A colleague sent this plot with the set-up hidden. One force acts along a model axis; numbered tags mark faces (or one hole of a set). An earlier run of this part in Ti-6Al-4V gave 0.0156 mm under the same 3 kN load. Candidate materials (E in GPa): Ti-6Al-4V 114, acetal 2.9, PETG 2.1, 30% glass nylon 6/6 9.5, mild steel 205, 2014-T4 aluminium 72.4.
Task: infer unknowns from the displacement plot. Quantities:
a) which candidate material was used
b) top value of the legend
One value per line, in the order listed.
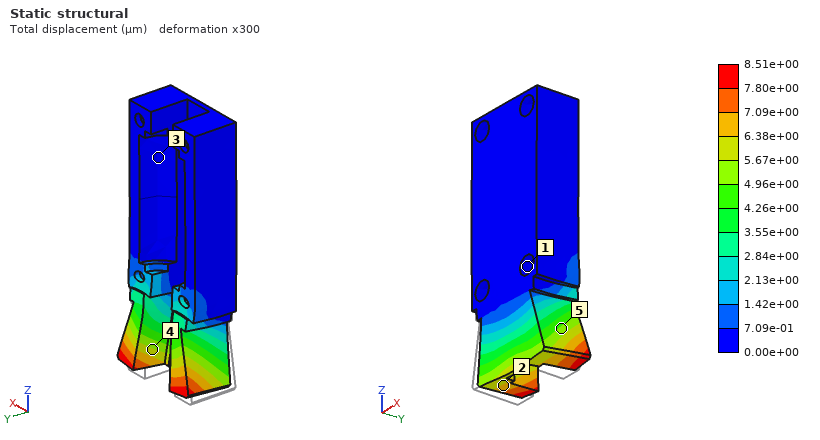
mild steel
8.51e+00 µm
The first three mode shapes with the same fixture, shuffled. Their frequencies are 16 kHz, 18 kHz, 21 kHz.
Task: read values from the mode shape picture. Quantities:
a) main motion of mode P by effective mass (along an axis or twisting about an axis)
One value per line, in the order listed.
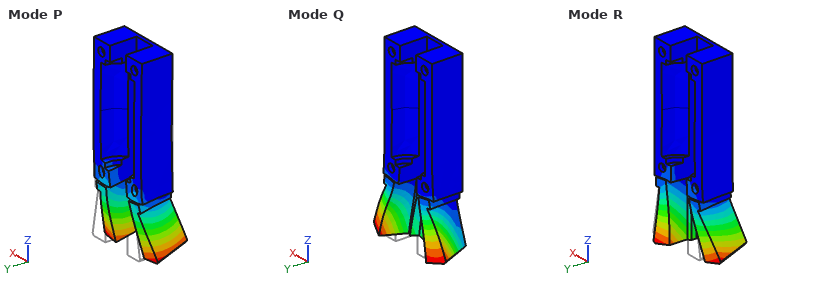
along Y
